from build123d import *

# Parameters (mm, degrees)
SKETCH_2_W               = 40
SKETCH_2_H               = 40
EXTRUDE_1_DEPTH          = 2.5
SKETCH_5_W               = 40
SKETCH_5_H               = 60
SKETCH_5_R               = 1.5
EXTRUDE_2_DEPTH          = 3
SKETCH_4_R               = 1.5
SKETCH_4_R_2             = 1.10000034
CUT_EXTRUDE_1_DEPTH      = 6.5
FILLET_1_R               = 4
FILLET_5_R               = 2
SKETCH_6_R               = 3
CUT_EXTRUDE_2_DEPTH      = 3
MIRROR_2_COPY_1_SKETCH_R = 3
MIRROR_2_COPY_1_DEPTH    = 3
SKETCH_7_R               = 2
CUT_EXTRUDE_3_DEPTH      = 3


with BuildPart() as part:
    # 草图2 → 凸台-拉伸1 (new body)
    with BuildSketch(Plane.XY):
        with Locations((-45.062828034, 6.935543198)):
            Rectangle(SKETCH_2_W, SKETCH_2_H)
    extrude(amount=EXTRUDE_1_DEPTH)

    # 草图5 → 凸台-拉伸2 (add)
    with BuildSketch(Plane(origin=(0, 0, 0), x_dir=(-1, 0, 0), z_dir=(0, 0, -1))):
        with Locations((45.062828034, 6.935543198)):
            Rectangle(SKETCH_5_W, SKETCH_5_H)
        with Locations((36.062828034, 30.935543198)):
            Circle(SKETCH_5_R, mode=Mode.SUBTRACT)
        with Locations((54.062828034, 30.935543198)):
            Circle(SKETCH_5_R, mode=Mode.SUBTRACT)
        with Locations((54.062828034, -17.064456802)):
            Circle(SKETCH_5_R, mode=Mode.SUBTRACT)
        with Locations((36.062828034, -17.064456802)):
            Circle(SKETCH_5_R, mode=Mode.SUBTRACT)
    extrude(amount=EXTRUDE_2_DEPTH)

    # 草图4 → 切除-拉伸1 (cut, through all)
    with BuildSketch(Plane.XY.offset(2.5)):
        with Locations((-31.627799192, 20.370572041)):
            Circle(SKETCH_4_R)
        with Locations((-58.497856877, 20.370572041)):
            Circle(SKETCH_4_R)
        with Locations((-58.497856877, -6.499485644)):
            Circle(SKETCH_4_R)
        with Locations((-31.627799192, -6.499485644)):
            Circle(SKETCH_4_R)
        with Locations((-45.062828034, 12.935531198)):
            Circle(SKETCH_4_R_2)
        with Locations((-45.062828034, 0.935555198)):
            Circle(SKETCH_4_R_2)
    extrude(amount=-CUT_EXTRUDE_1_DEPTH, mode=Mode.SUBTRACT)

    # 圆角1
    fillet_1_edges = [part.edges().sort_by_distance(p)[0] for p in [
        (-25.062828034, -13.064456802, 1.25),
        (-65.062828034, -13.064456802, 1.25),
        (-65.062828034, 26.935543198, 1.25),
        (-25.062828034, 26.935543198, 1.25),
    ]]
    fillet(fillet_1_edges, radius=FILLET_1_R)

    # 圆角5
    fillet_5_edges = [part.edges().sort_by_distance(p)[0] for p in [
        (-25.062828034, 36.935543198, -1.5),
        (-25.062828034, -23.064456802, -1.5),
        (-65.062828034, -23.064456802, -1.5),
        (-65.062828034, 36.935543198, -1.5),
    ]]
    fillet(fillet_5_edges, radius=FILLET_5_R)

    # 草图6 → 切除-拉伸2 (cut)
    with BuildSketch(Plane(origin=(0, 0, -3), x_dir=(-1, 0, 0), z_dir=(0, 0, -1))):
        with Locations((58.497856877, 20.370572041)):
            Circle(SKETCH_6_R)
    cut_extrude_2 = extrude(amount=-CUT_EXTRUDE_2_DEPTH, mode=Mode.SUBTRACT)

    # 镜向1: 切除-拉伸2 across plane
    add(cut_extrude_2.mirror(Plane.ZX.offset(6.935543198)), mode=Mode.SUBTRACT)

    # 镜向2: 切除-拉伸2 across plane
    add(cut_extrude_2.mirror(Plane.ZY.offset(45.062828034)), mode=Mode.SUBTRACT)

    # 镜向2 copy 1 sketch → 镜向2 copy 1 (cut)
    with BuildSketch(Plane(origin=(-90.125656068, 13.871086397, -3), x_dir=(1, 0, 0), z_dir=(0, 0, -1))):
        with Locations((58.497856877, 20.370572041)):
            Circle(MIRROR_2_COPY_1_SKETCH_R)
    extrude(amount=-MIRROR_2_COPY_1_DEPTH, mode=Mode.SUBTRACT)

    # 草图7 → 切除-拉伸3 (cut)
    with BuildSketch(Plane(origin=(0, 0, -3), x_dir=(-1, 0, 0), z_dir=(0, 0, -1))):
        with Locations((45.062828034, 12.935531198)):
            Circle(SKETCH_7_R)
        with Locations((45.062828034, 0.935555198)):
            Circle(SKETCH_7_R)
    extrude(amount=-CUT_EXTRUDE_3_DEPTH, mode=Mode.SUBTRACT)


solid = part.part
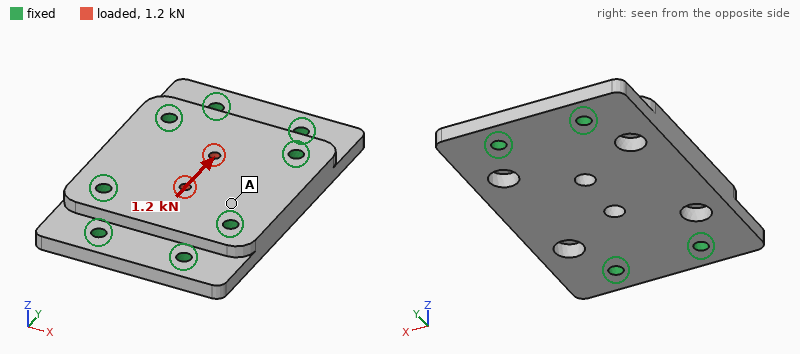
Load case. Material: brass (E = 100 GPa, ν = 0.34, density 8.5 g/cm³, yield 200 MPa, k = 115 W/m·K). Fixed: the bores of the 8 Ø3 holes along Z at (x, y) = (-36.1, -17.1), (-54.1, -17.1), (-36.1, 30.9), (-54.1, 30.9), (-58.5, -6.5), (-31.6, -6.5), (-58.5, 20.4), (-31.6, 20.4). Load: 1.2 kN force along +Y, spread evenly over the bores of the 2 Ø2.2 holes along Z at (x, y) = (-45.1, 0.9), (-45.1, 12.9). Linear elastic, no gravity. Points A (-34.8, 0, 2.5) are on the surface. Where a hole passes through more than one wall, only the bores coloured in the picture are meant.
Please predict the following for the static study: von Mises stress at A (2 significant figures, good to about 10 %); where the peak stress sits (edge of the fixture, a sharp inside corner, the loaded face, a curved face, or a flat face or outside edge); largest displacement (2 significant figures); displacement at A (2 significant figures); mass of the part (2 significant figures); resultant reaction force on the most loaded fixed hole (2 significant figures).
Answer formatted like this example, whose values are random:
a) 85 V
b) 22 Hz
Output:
a) 4.7 MPa
b) the loaded face
c) 2.1 µm
d) 0.40 µm
e) 90 g
f) 170 N
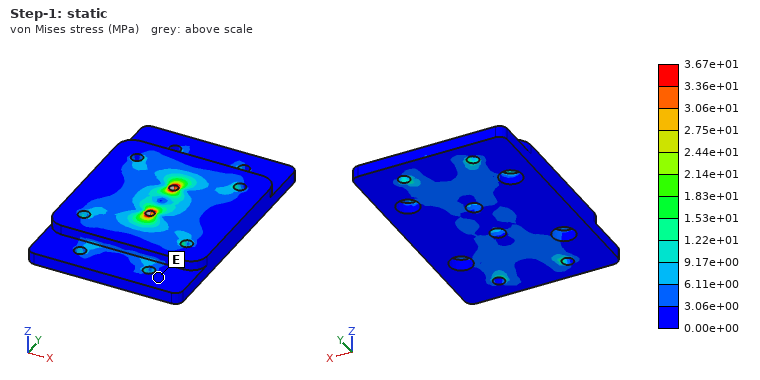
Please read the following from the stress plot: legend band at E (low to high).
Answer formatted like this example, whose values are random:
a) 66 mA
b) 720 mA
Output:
a) 0.00e+00 to 3.06e+00 MPa
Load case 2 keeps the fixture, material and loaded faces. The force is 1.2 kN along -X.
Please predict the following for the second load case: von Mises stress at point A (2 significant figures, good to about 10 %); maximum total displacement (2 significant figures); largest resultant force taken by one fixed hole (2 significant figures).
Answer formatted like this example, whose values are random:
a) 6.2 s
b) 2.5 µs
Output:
a) 6.6 MPa
b) 2.2 µm
c) 260 N
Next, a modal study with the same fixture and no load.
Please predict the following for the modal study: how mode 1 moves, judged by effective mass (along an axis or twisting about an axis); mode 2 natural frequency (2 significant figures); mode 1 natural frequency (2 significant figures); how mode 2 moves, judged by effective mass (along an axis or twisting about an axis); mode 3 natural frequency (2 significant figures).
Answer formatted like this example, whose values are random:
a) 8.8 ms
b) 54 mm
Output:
a) along Z
b) 17 kHz
c) 13 kHz
d) twisting about Y
e) 19 kHz
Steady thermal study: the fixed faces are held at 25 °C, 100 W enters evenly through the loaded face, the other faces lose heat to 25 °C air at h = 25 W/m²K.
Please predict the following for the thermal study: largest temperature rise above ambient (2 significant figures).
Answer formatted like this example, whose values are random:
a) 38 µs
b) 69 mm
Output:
a) 74 K
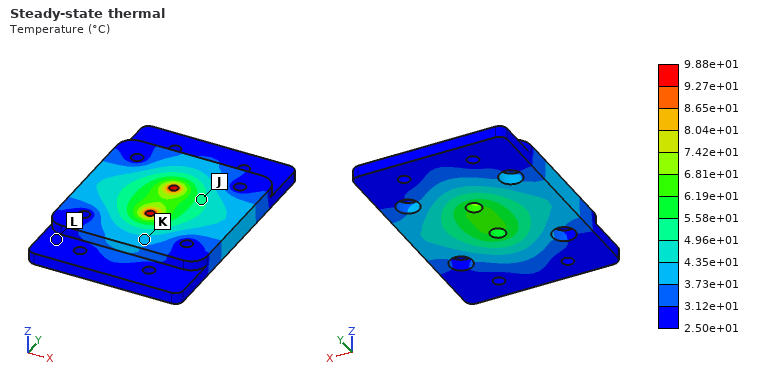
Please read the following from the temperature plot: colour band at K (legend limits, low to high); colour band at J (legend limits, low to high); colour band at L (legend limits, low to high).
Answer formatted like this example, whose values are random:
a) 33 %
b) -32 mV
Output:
a) 3.73e+01 to 4.35e+01 °C
b) 4.96e+01 to 5.58e+01 °C
c) 2.50e+01 to 3.12e+01 °C
